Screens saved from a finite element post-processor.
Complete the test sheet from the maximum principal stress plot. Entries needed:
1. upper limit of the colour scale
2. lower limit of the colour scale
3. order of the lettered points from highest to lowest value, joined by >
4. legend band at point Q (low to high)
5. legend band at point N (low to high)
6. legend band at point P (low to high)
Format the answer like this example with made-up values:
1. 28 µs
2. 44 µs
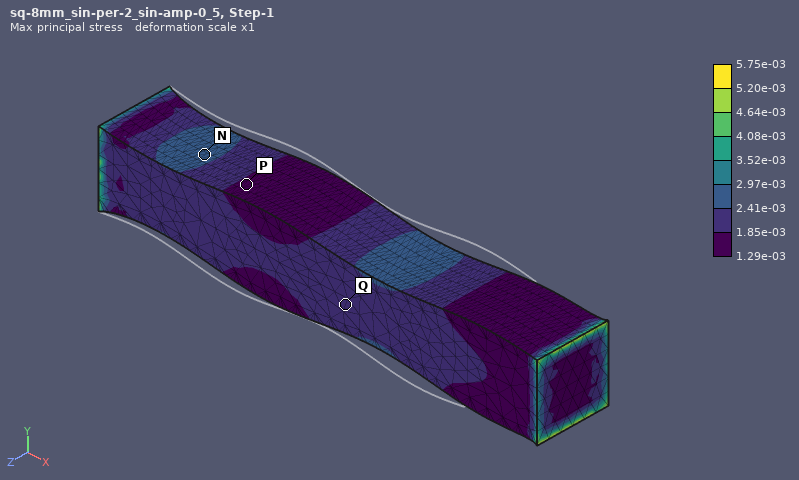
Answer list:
1. 5.75e-03
2. 1.29e-03
3. N > Q > P
4. 1.85e-03 to 2.41e-03
5. 2.41e-03 to 2.97e-03
6. 1.29e-03 to 1.85e-03
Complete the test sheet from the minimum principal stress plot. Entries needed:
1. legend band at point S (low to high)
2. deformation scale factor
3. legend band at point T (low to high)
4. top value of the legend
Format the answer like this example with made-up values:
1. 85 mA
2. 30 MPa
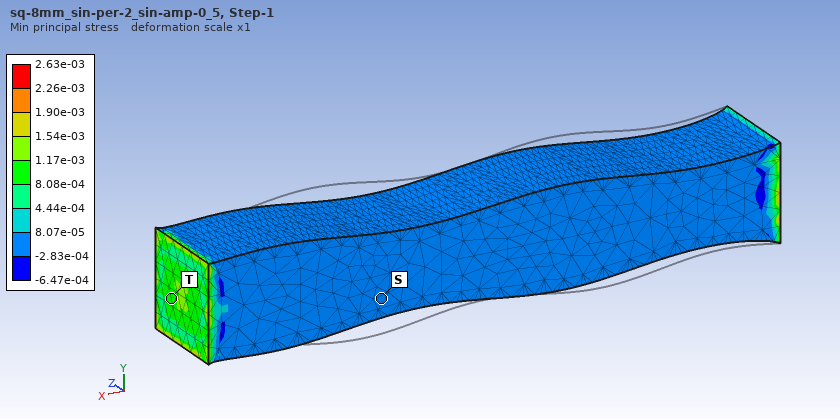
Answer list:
1. -2.83e-04 to 8.07e-05
2. 1
3. 8.08e-04 to 1.17e-03
4. 2.63e-03
